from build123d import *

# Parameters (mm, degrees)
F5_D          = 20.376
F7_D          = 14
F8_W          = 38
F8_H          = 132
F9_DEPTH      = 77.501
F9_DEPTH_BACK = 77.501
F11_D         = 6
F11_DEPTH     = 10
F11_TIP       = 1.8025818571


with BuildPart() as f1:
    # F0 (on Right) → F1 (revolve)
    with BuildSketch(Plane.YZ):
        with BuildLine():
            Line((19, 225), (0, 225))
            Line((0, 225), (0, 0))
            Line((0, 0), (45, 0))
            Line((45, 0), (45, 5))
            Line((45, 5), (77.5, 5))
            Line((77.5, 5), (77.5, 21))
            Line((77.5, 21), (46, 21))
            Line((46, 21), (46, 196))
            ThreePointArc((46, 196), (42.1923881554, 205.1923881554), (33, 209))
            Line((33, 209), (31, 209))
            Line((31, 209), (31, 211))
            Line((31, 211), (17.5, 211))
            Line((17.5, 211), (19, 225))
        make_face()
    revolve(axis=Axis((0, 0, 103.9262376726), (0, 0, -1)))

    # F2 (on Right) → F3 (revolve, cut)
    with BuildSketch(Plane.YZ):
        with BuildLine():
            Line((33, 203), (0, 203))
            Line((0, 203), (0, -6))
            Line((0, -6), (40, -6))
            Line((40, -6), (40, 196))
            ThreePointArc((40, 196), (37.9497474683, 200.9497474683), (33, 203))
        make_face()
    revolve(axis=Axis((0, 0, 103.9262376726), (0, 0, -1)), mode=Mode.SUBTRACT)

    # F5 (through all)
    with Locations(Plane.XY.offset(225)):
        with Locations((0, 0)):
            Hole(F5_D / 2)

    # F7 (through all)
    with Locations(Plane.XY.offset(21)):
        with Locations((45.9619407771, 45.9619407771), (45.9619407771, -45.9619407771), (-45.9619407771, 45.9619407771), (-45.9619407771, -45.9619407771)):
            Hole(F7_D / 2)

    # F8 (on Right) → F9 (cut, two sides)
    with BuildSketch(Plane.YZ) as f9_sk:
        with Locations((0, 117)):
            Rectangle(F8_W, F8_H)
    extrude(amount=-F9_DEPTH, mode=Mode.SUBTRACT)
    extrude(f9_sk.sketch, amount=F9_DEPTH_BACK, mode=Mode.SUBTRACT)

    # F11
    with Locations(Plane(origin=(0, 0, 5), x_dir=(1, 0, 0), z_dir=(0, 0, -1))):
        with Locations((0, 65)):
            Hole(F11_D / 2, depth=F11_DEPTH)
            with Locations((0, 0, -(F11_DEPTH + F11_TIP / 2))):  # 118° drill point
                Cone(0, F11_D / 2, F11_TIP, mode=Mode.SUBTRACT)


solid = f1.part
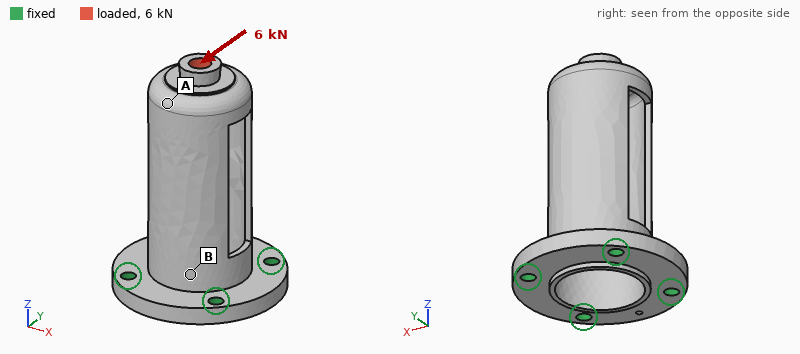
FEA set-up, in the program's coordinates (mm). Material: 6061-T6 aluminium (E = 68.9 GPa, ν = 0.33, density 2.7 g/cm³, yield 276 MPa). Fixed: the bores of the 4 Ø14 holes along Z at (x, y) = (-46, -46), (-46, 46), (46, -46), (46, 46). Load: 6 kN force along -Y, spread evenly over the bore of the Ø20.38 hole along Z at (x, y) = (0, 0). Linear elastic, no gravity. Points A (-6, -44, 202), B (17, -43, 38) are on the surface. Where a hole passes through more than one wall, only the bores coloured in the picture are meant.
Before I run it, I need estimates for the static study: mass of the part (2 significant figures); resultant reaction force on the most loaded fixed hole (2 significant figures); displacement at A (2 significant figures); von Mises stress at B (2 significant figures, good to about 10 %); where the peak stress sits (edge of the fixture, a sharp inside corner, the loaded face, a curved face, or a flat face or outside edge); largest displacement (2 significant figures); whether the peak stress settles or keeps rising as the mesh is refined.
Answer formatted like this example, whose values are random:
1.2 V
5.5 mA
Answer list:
1.3 kg
7.4 kN
1.1 mm
61 MPa
a sharp inside corner
1.2 mm
keeps rising
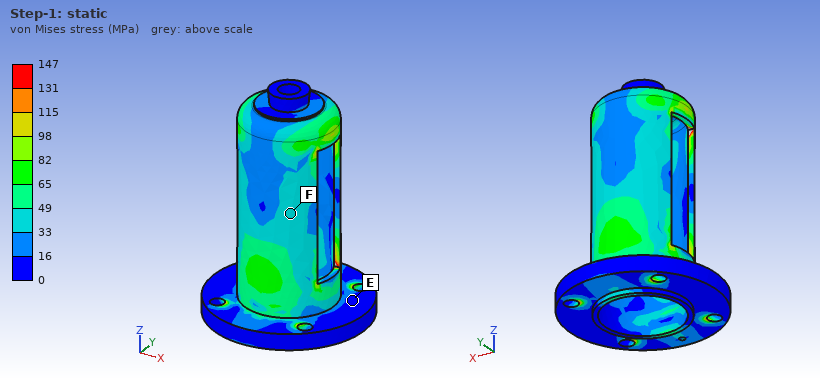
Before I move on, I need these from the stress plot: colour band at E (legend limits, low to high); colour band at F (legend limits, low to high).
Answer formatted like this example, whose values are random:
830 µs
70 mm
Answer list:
0 to 16 MPa
33 to 49 MPa
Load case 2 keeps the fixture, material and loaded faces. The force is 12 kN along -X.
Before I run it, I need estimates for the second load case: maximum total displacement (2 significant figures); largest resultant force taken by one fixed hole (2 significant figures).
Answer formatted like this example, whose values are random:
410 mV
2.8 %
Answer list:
1.0 mm
16 kN
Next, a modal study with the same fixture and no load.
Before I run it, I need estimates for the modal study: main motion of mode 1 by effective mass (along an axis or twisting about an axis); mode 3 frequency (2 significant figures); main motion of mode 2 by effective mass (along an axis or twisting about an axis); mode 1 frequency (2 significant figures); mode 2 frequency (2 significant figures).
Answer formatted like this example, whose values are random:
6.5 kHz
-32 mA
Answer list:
along Y
1800 Hz
along X
640 Hz
1100 Hz
